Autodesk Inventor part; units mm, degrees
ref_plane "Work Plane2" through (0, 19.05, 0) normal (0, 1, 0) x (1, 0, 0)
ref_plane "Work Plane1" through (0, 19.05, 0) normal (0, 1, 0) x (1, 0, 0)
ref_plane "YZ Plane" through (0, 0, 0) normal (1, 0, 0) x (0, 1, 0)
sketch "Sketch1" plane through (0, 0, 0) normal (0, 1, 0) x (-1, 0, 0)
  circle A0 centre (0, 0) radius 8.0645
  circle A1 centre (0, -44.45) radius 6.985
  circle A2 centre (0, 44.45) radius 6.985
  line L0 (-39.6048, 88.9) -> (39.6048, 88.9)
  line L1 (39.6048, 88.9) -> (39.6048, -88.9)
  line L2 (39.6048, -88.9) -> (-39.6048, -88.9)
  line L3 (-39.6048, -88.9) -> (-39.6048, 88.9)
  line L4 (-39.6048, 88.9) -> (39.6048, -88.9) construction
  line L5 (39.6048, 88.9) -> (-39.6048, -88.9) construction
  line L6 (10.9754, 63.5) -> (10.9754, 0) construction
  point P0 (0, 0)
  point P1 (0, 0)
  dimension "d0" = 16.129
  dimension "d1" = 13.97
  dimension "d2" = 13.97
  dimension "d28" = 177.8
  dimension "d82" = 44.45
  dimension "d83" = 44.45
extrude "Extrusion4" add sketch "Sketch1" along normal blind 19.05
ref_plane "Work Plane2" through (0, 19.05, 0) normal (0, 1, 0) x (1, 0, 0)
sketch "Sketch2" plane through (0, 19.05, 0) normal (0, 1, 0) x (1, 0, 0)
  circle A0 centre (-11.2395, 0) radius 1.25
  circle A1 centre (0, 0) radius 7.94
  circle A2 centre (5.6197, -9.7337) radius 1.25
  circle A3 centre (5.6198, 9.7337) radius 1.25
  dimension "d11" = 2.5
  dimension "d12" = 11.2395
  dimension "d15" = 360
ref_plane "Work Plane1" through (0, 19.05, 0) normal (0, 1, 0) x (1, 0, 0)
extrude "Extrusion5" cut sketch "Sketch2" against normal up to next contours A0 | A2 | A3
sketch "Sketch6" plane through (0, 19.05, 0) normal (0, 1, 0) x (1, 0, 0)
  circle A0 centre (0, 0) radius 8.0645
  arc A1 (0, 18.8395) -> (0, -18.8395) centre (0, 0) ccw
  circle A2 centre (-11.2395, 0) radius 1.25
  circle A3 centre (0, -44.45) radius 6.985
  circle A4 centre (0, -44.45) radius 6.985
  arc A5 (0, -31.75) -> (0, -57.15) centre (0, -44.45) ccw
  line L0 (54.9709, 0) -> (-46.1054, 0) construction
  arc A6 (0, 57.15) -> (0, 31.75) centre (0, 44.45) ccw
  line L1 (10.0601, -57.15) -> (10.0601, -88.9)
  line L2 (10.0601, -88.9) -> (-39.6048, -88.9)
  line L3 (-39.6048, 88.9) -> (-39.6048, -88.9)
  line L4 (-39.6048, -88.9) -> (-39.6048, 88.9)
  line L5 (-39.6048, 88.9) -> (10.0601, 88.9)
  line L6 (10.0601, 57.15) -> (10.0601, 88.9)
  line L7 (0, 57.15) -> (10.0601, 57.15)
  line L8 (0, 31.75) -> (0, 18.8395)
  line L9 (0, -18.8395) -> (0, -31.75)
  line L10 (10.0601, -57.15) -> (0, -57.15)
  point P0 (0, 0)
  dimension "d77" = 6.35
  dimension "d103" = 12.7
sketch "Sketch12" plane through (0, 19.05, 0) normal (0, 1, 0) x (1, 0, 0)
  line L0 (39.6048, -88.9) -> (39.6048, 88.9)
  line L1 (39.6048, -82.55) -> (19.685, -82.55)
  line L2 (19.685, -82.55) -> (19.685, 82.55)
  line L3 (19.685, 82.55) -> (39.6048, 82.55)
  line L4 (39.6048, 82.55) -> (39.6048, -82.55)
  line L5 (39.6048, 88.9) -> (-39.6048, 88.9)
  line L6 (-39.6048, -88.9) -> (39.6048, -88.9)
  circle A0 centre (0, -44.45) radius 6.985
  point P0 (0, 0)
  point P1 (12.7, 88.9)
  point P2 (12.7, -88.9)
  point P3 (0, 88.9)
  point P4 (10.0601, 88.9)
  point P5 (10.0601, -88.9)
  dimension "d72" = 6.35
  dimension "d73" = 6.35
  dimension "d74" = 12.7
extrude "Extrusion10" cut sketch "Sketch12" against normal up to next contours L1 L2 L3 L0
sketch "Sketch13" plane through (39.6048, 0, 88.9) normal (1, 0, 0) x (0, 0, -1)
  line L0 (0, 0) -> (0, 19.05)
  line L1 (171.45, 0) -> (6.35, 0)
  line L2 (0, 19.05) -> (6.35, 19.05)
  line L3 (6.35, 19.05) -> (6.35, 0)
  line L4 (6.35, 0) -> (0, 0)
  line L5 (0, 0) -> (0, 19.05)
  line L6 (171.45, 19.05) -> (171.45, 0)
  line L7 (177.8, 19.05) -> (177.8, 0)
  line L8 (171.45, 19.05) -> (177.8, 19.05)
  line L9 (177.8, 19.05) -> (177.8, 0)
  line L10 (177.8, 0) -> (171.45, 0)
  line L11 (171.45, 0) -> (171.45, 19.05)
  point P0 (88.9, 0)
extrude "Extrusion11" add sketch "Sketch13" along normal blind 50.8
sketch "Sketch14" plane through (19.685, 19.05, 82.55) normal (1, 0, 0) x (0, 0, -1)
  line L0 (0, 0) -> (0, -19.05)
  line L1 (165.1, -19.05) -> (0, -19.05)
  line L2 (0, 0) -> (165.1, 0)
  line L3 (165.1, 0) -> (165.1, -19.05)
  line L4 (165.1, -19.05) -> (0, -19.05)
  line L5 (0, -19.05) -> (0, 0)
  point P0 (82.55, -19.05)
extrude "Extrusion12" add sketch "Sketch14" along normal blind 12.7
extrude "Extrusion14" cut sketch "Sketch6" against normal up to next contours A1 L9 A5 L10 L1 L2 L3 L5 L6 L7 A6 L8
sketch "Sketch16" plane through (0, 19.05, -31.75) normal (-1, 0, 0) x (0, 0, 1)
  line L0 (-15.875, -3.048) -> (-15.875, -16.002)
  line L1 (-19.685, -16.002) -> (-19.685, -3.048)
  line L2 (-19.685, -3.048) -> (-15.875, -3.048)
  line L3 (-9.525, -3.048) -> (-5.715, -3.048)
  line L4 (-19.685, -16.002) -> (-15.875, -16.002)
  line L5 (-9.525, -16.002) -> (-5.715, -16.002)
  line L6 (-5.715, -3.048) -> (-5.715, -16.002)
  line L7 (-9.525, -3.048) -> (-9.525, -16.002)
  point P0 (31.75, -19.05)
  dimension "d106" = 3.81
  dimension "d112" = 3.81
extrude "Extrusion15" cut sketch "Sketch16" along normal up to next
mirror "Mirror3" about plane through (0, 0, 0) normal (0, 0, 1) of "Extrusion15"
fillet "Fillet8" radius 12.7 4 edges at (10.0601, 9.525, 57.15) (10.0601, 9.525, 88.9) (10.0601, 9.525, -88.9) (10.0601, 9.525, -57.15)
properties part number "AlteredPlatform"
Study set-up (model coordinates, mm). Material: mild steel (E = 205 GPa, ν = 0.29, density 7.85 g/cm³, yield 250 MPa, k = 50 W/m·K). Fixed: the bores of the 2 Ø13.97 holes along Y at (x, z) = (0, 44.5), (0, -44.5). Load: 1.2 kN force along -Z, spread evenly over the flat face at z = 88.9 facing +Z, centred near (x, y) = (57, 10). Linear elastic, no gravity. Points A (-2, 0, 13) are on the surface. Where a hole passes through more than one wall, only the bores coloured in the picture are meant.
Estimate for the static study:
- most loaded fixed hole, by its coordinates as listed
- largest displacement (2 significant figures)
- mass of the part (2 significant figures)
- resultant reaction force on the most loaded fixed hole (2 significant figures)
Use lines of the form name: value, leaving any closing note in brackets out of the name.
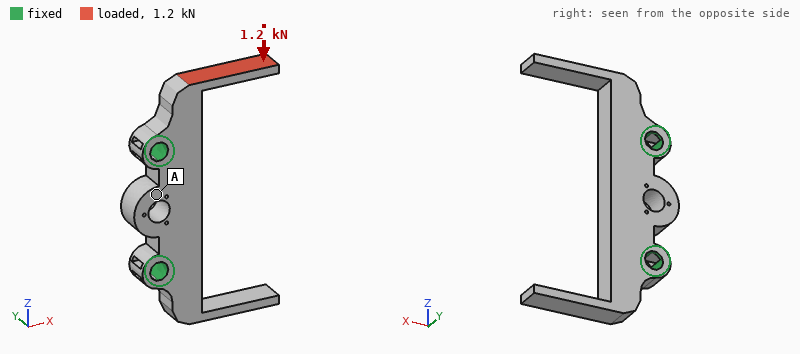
most loaded fixed hole, by its coordinates as listed: (0, -44.5)
largest displacement: 0.39 mm
mass of the part: 940 g
resultant reaction force on the most loaded fixed hole: 1.1 kN
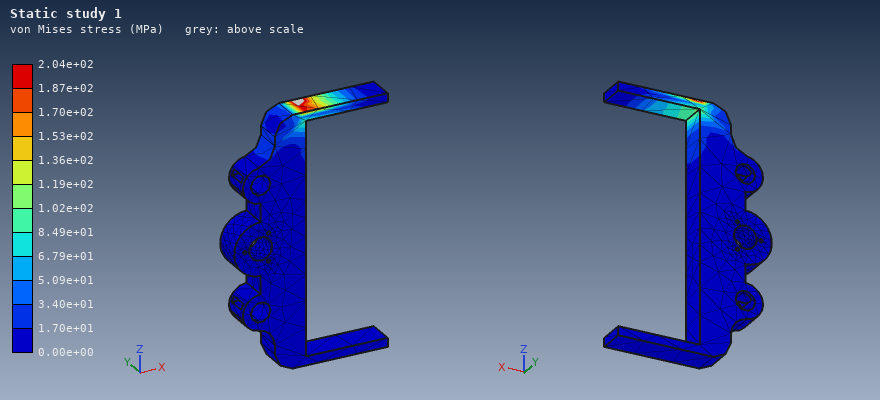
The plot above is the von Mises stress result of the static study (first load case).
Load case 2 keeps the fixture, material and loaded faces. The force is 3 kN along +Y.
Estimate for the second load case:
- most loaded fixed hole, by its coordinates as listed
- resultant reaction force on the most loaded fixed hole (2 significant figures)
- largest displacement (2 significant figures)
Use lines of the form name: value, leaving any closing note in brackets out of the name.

most loaded fixed hole, by its coordinates as listed: (0, 44.5)
resultant reaction force on the most loaded fixed hole: 3.5 kN
largest displacement: 0.32 mm
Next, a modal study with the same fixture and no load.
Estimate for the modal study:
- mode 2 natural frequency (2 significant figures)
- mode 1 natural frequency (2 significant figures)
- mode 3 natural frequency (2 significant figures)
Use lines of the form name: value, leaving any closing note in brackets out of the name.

mode 2 natural frequency: 1400 Hz
mode 1 natural frequency: 1400 Hz
mode 3 natural frequency: 2300 Hz
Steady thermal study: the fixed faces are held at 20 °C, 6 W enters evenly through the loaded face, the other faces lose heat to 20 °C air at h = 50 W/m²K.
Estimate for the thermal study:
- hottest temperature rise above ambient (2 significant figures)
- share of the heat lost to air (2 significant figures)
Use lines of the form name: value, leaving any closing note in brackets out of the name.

hottest temperature rise above ambient: 24 K
share of the heat lost to air: 46 %
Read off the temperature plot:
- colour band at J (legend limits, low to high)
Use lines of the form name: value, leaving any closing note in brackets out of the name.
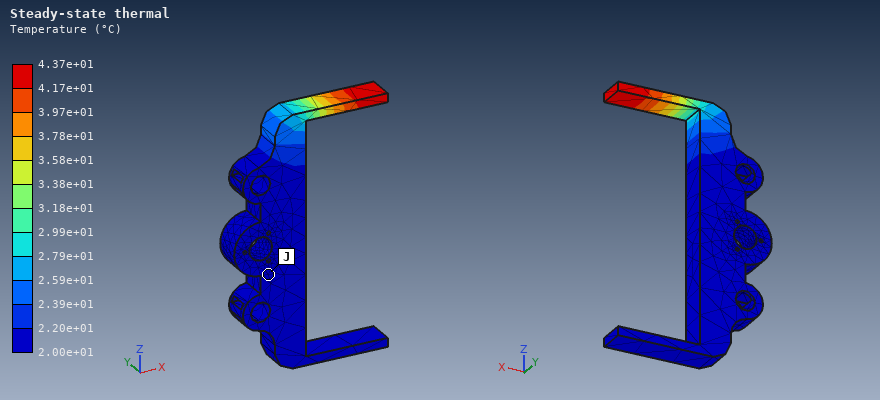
colour band at J: 2.00e+01 to 2.20e+01 °C
